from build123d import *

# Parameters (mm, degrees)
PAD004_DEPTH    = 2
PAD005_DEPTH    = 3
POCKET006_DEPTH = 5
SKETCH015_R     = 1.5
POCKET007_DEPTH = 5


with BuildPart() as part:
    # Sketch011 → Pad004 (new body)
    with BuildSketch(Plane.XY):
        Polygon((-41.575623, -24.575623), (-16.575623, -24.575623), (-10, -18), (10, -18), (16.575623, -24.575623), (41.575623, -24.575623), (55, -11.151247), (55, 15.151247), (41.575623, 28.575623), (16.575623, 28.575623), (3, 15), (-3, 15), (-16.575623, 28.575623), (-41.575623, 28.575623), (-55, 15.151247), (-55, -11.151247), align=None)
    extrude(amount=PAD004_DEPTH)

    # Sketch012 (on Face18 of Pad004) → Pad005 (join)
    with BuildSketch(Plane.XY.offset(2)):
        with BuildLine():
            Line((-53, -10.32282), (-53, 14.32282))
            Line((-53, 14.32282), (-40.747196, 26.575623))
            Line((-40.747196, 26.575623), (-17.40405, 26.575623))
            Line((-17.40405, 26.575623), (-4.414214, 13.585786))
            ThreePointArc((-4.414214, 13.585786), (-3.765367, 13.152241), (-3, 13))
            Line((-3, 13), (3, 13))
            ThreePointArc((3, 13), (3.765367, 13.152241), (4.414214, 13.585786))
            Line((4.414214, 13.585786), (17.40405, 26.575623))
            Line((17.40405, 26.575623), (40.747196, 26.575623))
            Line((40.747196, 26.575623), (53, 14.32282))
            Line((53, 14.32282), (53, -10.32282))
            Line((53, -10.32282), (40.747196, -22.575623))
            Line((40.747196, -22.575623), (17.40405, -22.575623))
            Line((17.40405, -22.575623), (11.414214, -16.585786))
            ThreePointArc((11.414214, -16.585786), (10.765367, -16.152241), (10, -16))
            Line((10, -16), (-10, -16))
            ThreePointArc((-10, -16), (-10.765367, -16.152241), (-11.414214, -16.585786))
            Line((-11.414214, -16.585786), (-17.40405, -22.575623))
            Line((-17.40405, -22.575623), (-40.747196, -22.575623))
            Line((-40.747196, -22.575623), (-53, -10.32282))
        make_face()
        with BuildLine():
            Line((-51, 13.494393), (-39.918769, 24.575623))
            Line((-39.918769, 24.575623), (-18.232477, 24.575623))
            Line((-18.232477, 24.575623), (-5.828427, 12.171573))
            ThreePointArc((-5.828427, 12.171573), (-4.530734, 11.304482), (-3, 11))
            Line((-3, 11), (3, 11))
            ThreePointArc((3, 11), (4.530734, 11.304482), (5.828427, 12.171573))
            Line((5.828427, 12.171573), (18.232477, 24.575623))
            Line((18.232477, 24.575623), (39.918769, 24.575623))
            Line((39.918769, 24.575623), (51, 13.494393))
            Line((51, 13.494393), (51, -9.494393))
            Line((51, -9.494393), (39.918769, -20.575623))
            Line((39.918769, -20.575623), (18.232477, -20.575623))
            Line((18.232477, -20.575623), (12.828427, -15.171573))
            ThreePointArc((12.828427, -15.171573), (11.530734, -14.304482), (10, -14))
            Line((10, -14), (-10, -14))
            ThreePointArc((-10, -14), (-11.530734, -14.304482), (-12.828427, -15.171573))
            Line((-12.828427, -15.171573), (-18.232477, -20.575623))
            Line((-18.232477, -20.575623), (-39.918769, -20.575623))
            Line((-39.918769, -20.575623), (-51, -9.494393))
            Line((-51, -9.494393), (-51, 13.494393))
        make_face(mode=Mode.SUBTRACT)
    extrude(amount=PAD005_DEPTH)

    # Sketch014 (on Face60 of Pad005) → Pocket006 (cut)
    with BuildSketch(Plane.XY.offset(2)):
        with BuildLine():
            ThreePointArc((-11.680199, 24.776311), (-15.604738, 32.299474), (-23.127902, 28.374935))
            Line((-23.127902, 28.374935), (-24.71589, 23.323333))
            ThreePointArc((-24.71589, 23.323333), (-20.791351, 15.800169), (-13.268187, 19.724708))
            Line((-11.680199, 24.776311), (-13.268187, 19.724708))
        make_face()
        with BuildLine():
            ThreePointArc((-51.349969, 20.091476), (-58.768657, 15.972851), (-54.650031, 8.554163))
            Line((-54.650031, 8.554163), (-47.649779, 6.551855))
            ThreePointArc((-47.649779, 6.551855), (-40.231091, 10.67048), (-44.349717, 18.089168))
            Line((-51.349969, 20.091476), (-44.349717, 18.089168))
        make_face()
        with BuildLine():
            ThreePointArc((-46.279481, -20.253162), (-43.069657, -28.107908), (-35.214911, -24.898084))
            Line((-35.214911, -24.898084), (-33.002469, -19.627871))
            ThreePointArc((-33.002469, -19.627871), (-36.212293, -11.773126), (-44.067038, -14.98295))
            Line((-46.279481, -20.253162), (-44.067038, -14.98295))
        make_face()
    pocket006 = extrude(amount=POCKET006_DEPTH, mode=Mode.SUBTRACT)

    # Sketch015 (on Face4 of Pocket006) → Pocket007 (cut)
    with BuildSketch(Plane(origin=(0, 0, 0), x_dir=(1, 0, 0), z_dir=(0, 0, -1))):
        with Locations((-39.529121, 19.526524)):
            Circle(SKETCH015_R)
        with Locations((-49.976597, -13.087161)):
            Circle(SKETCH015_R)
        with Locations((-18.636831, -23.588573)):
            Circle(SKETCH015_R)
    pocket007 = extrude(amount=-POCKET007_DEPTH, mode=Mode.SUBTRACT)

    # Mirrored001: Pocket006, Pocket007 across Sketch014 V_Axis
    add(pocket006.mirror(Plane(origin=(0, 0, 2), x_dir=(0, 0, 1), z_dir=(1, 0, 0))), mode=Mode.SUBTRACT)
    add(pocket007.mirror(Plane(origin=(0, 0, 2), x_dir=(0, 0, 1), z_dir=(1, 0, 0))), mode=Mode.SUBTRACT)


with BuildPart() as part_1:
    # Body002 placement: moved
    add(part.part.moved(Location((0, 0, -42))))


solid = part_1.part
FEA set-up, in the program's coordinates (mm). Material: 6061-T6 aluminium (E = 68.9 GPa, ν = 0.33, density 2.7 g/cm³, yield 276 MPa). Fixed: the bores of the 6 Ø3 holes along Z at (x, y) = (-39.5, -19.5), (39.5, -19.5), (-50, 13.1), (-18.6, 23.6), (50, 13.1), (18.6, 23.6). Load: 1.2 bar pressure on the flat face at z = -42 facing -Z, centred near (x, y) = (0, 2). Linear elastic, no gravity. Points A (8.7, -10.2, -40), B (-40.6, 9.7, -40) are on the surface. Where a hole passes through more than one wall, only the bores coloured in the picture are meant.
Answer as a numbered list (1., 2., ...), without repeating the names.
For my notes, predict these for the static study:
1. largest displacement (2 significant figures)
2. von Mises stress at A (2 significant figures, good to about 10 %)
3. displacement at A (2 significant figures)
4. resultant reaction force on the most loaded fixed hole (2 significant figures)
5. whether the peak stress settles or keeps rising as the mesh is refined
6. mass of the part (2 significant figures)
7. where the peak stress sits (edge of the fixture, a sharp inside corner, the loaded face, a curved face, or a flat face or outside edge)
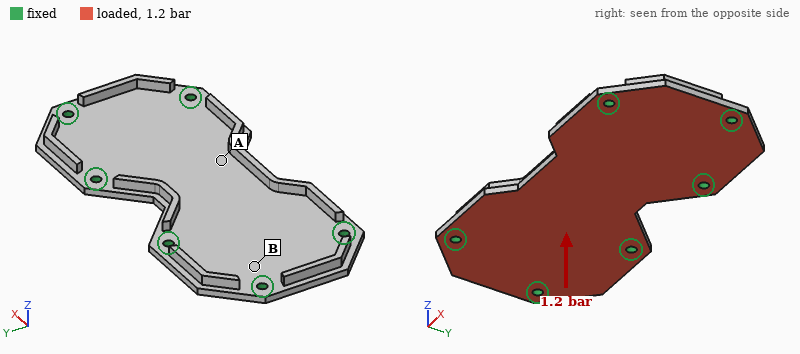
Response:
1. 0.12 mm
2. 20 MPa
3. 0.11 mm
4. 140 N
5. keeps rising
6. 30 g
7. edge of the fixture
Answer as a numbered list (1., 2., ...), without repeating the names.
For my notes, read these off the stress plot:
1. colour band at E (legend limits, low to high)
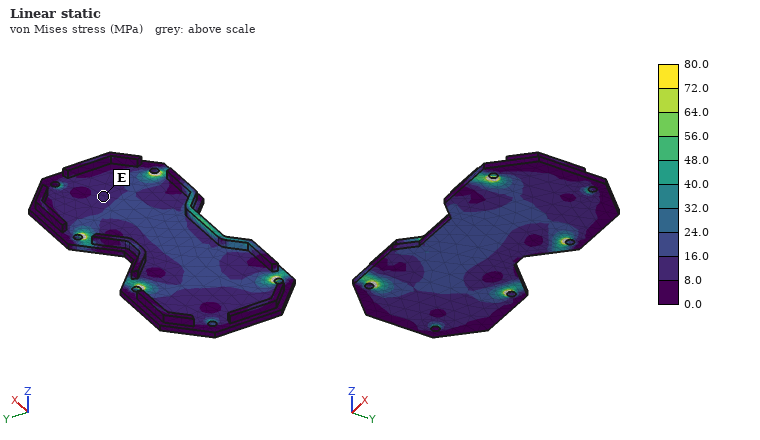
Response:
1. 8.0 to 16.0 MPa
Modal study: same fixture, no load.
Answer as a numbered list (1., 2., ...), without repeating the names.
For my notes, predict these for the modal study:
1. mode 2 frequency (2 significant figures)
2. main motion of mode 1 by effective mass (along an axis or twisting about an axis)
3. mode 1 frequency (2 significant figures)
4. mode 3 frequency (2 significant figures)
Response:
1. 5300 Hz
2. along Z
3. 2400 Hz
4. 5500 Hz
